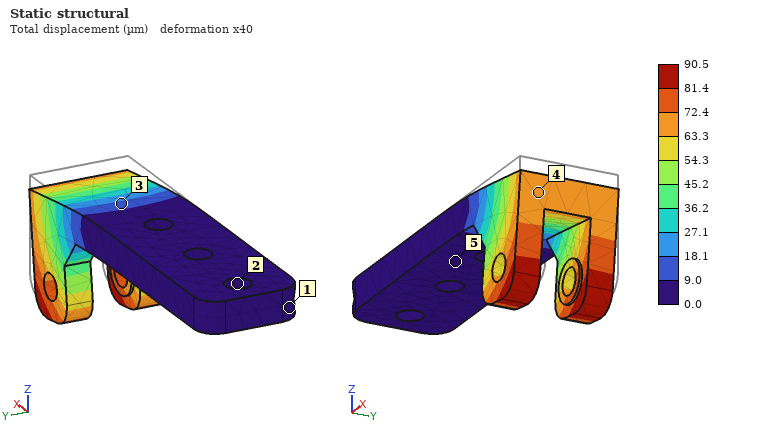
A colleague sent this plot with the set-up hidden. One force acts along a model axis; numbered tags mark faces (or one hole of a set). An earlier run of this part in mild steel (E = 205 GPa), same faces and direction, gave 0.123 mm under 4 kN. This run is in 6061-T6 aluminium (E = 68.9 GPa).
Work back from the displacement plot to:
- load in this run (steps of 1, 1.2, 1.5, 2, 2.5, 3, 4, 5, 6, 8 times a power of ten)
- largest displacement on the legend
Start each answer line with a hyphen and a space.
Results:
- 1 kN
- 90.5 µm
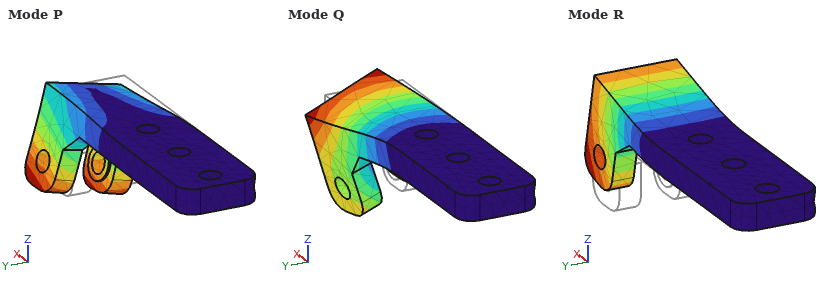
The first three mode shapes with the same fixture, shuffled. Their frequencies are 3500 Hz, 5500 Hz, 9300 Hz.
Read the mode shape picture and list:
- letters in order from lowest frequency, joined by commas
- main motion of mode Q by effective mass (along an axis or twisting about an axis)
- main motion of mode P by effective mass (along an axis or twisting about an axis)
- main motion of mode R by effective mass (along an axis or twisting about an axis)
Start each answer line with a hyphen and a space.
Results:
- R, P, Q
- along Y
- along Y
- along Z
